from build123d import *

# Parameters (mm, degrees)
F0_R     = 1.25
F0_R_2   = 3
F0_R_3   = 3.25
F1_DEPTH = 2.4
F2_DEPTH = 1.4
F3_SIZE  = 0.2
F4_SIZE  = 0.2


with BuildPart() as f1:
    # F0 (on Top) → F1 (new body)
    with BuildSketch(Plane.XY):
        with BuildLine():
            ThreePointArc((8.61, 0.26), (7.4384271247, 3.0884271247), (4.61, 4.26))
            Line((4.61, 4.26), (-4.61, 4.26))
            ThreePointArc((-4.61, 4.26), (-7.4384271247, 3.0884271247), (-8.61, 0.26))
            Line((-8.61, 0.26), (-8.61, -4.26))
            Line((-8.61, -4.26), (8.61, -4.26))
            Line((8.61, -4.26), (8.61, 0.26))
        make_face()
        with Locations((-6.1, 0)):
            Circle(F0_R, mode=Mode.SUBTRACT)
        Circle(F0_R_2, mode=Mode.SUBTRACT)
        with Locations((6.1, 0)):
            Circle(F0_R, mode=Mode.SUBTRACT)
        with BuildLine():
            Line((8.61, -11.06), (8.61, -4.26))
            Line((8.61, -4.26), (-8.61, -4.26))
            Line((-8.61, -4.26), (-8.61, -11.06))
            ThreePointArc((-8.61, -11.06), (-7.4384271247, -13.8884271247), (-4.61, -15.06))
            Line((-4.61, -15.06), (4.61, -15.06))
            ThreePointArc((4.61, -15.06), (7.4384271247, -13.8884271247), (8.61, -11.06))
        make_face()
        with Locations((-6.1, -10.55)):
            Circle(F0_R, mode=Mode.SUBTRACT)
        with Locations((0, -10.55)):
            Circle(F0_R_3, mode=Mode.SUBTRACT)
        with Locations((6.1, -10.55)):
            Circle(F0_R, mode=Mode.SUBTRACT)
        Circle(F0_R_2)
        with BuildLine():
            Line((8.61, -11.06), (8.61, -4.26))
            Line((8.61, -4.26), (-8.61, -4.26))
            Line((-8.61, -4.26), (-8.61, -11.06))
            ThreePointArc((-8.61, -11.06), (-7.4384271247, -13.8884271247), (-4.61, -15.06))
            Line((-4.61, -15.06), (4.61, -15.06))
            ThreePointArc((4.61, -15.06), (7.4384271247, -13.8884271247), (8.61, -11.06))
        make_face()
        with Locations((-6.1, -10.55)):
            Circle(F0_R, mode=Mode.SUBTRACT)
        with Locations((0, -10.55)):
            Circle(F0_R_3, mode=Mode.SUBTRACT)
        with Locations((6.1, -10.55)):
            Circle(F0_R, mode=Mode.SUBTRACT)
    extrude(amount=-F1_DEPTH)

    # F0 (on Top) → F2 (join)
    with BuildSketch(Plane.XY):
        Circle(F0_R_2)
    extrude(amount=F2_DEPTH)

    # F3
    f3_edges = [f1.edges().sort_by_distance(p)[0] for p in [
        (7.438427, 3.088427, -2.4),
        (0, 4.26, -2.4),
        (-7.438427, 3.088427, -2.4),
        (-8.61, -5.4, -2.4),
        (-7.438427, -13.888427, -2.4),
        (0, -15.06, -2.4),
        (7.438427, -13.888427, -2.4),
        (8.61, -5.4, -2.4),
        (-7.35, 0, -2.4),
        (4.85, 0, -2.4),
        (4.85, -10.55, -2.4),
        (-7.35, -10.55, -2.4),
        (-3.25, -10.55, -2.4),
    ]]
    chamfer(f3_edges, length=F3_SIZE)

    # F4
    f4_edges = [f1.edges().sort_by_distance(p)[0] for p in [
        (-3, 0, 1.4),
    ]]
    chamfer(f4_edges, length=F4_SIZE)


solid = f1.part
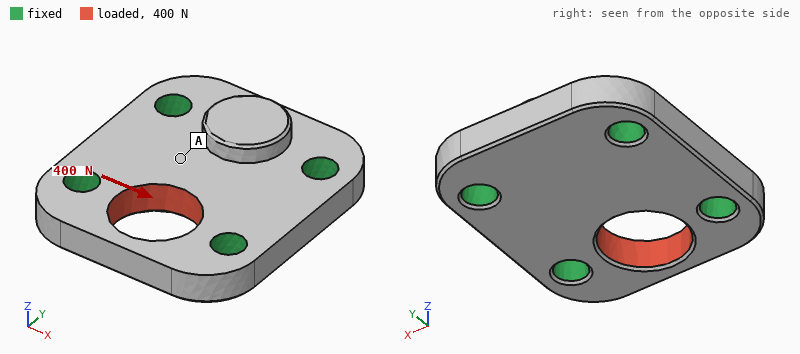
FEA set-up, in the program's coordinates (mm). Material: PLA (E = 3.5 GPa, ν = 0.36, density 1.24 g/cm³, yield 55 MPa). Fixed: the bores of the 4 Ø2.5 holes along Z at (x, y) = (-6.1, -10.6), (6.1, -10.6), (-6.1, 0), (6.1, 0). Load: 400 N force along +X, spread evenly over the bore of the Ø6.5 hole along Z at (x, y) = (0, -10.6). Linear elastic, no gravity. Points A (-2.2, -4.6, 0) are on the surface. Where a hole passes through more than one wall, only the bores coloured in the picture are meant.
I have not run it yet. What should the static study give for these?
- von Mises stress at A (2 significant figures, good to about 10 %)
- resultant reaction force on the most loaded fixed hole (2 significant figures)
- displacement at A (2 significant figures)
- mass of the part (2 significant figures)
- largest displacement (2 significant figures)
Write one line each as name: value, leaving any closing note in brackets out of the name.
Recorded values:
von Mises stress at A: 3.1 MPa
resultant reaction force on the most loaded fixed hole: 170 N
displacement at A: 5.4 µm
mass of the part: 0.84 g
largest displacement: 34 µm
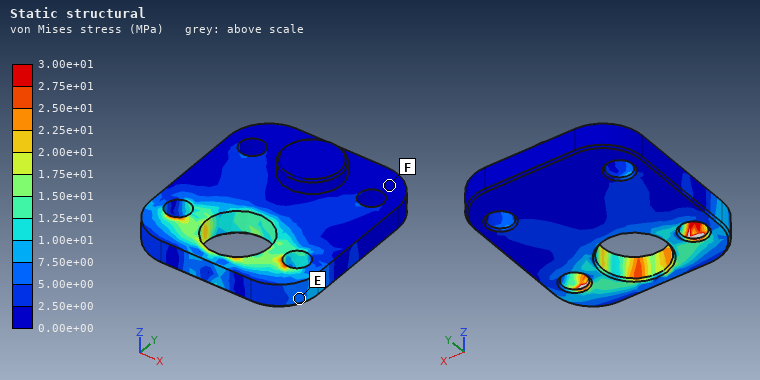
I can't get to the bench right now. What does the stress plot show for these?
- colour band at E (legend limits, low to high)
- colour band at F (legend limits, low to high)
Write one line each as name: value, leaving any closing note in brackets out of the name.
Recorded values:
colour band at E: 5.00e+00 to 7.50e+00 MPa
colour band at F: 0.00e+00 to 2.50e+00 MPa
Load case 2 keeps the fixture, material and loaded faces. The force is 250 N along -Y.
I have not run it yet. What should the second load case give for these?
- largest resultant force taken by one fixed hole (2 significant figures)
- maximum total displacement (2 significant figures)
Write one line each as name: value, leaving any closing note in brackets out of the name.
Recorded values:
largest resultant force taken by one fixed hole: 93 N
maximum total displacement: 45 µm
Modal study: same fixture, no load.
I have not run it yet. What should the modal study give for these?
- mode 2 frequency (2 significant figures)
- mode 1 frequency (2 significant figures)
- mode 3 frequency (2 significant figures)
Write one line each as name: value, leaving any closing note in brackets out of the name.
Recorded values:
mode 2 frequency: 23 kHz
mode 1 frequency: 22 kHz
mode 3 frequency: 23 kHz
